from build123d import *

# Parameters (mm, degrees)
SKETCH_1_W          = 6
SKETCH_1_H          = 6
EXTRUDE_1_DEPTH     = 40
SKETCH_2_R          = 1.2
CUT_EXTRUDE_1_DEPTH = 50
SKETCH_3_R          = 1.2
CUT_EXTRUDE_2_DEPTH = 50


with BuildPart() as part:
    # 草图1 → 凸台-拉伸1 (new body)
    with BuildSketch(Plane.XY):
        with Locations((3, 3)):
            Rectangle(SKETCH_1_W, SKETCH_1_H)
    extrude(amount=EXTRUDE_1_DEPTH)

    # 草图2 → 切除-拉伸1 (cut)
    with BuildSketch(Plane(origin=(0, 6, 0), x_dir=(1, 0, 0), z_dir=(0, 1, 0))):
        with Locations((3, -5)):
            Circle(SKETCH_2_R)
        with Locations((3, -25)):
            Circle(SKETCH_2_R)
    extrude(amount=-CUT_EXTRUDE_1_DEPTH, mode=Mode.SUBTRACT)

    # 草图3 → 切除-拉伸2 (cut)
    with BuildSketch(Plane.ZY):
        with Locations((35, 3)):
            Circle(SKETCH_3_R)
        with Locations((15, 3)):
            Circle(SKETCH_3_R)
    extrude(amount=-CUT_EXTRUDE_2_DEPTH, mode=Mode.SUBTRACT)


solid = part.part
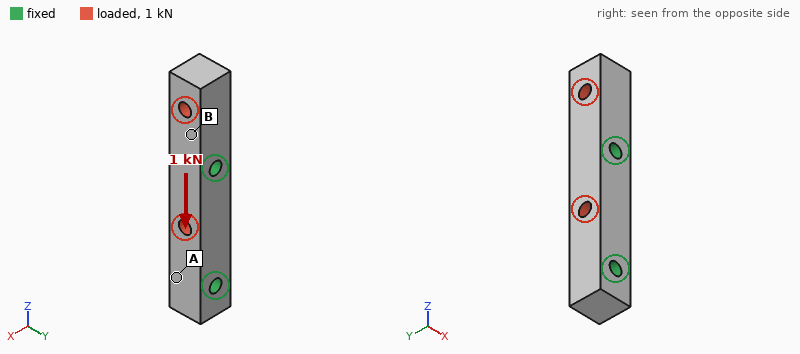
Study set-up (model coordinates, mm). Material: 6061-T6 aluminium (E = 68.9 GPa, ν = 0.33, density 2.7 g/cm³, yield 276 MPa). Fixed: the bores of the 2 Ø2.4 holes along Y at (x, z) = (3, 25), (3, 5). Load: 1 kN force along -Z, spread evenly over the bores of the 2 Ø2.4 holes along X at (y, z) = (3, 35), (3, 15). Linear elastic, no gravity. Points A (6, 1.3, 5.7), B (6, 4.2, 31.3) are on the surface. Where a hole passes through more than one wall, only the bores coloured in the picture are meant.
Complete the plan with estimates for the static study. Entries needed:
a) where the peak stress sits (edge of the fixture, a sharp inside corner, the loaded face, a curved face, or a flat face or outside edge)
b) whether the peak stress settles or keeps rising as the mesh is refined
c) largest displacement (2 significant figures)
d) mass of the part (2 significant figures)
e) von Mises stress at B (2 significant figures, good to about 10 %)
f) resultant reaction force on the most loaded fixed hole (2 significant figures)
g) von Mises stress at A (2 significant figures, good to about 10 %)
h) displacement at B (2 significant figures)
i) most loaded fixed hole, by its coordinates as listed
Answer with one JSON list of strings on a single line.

["edge of the fixture", "keeps rising", "2.6 µm", "3.6 g", "14 MPa", "740 N", "3.6 MPa", "1.3 µm", "(3, 25)"]
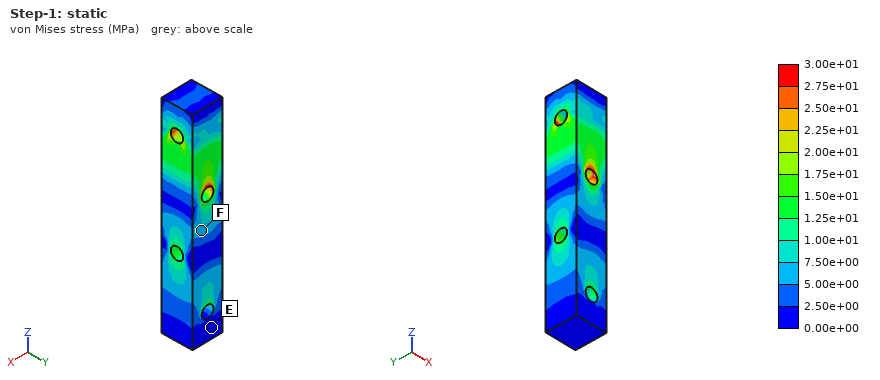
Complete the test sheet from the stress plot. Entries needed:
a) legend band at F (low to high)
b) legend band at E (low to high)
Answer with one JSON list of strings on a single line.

["5.00e+00 to 7.50e+00 MPa", "0.00e+00 to 2.50e+00 MPa"]
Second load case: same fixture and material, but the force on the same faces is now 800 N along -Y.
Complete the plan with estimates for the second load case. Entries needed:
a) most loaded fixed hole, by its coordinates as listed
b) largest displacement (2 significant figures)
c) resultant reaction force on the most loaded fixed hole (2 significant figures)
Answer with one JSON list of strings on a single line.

["(3, 25)", "35 µm", "610 N"]
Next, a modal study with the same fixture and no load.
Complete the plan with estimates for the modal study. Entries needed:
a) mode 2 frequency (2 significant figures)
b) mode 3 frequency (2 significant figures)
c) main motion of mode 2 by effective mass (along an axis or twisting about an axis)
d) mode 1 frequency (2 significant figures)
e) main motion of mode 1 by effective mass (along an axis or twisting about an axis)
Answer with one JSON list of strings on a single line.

["21 kHz", "48 kHz", "along Y", "18 kHz", "along X"]
